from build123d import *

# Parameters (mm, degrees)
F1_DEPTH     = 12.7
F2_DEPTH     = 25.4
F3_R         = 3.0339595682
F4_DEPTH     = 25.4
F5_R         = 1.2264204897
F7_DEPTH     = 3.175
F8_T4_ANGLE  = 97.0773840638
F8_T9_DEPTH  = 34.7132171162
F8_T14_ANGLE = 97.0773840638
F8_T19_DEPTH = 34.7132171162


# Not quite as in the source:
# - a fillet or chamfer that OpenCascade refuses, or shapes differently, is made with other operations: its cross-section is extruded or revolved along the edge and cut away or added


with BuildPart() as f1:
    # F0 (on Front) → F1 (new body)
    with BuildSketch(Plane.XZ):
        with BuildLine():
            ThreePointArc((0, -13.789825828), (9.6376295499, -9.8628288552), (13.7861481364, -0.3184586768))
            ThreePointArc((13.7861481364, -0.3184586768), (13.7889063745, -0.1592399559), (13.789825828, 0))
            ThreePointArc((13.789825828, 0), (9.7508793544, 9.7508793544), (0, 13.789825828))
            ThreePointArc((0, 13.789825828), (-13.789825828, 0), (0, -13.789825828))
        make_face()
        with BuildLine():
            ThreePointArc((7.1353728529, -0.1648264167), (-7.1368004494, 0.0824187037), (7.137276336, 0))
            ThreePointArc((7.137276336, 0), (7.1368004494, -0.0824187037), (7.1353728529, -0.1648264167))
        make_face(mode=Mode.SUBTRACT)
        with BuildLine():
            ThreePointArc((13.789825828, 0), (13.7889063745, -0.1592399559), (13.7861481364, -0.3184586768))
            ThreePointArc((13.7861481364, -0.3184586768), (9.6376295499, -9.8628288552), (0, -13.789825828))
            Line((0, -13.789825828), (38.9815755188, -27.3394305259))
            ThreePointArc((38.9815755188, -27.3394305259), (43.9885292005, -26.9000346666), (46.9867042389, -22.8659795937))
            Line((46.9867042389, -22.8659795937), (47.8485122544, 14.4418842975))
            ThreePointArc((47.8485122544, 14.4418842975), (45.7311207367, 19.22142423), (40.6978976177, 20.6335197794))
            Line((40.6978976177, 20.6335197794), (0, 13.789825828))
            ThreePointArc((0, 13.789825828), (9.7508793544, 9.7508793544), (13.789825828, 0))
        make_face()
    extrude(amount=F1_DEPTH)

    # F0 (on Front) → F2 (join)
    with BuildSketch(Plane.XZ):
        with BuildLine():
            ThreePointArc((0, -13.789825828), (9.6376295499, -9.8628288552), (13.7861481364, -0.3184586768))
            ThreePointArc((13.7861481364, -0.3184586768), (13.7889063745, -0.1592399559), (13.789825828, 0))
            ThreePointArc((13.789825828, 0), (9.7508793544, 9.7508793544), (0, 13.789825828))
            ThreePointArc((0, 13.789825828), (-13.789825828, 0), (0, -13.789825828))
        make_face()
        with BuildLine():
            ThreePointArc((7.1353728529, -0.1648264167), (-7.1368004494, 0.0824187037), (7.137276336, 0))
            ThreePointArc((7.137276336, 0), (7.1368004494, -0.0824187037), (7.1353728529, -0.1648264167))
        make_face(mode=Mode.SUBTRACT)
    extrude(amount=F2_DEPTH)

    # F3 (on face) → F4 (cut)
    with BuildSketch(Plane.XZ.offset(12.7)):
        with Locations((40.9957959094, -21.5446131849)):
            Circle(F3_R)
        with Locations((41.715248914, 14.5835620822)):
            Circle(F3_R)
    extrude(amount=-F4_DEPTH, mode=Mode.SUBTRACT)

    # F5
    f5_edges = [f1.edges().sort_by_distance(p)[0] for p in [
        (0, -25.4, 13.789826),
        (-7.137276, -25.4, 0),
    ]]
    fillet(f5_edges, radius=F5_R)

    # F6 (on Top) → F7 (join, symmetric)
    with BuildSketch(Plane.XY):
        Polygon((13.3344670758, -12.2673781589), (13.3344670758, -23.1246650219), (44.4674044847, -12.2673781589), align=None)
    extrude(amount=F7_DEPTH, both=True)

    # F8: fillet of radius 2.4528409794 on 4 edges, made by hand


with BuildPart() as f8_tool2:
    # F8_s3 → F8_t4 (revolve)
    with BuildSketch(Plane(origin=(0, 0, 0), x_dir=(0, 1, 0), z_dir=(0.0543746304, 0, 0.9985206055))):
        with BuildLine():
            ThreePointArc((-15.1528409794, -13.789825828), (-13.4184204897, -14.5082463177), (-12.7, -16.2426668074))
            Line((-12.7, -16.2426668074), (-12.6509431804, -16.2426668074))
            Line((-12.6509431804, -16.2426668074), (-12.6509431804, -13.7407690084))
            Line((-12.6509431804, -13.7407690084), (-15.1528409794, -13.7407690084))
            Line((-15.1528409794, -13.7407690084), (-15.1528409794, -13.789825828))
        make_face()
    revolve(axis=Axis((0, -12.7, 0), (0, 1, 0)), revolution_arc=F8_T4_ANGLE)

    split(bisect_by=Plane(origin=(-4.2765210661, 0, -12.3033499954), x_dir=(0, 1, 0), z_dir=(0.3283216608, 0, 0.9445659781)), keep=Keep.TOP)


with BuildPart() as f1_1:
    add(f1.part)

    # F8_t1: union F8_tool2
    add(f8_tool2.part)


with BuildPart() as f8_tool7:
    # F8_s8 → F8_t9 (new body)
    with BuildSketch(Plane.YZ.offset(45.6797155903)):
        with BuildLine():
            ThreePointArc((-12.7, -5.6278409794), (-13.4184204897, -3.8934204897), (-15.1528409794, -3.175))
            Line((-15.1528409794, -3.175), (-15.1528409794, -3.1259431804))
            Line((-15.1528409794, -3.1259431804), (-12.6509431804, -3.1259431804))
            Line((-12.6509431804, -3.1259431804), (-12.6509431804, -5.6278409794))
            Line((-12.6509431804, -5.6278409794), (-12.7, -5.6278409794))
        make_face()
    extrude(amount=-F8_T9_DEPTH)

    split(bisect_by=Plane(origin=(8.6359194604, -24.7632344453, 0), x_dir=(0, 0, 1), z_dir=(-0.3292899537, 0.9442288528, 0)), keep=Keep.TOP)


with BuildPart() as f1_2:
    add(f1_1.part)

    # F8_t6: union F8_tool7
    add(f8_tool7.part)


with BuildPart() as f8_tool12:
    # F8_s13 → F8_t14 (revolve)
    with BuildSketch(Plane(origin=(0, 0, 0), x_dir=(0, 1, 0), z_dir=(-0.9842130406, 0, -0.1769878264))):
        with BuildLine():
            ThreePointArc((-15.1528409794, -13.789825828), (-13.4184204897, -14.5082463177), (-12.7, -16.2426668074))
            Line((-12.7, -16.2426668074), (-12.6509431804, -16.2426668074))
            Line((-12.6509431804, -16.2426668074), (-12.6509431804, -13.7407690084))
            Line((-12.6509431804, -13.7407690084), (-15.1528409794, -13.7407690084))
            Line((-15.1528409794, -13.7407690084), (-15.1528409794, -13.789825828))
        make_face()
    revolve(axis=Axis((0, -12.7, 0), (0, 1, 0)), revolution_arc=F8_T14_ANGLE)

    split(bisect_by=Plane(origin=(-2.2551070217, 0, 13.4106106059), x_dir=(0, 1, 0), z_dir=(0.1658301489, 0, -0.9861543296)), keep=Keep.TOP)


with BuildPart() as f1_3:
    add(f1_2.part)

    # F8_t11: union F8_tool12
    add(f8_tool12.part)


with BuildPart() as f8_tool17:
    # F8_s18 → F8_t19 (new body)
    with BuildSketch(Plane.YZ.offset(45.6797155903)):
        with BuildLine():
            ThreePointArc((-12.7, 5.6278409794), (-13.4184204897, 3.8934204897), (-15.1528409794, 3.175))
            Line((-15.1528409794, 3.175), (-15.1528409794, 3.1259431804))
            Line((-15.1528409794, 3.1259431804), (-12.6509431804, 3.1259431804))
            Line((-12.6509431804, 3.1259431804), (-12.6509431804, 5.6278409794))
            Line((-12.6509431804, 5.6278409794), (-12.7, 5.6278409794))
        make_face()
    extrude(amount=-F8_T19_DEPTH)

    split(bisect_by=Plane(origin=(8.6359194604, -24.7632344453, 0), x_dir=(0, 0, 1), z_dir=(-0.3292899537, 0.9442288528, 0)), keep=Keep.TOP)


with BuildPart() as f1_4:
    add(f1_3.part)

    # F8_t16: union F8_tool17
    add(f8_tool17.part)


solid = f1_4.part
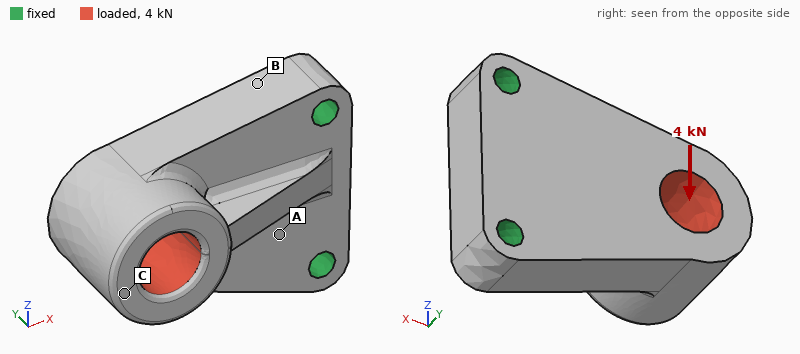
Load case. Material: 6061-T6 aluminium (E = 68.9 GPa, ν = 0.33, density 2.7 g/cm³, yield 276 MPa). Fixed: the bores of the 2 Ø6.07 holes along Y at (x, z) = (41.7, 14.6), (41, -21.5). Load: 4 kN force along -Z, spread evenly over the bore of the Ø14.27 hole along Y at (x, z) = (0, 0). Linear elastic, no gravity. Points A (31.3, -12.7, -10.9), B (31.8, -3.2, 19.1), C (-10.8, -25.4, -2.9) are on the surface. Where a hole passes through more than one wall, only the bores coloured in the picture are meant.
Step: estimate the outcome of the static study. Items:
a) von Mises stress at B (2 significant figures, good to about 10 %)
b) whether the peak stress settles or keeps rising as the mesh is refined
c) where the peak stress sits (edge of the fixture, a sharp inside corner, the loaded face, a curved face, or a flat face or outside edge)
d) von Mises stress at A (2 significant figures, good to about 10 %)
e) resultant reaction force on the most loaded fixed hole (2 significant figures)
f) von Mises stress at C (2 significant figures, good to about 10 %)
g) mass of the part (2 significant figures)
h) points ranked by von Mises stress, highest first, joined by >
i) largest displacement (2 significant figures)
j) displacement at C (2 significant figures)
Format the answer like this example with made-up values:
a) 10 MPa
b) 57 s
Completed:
a) 35 MPa
b) keeps rising
c) edge of the fixture
d) 24 MPa
e) 4.9 kN
f) 4.9 MPa
g) 84 g
h) B > A > C
i) 57 µm
j) 56 µm
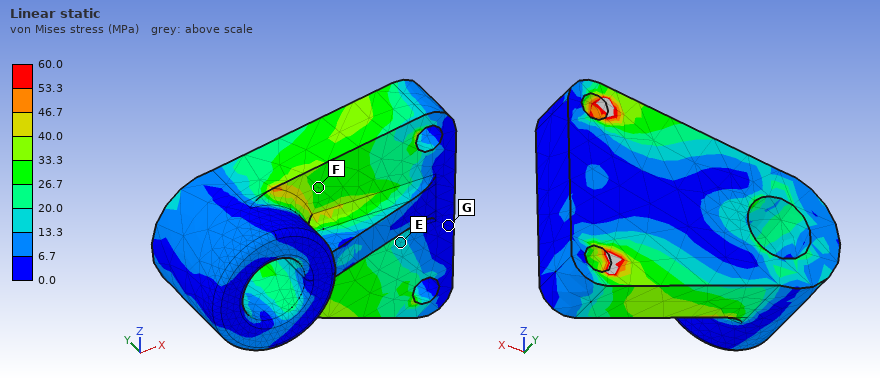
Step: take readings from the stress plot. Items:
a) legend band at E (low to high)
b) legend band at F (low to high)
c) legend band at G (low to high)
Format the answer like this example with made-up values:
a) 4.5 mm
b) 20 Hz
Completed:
a) 13.3 to 20.0 MPa
b) 26.7 to 33.3 MPa
c) 0.0 to 6.7 MPa
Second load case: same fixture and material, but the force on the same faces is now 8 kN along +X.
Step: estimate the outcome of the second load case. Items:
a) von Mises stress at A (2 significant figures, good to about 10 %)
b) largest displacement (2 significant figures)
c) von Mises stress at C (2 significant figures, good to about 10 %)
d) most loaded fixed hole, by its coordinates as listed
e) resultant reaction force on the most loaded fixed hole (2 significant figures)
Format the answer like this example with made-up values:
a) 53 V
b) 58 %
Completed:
a) 38 MPa
b) 0.13 mm
c) 10 MPa
d) (41.7, 14.6)
e) 5.0 kN
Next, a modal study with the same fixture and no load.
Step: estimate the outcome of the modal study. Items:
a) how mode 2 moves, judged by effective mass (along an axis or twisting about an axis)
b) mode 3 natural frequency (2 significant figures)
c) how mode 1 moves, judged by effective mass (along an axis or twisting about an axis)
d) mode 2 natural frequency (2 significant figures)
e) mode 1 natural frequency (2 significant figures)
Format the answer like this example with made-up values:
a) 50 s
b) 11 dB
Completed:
a) along Z
b) 12 kHz
c) along Y
d) 8400 Hz
e) 3400 Hz
